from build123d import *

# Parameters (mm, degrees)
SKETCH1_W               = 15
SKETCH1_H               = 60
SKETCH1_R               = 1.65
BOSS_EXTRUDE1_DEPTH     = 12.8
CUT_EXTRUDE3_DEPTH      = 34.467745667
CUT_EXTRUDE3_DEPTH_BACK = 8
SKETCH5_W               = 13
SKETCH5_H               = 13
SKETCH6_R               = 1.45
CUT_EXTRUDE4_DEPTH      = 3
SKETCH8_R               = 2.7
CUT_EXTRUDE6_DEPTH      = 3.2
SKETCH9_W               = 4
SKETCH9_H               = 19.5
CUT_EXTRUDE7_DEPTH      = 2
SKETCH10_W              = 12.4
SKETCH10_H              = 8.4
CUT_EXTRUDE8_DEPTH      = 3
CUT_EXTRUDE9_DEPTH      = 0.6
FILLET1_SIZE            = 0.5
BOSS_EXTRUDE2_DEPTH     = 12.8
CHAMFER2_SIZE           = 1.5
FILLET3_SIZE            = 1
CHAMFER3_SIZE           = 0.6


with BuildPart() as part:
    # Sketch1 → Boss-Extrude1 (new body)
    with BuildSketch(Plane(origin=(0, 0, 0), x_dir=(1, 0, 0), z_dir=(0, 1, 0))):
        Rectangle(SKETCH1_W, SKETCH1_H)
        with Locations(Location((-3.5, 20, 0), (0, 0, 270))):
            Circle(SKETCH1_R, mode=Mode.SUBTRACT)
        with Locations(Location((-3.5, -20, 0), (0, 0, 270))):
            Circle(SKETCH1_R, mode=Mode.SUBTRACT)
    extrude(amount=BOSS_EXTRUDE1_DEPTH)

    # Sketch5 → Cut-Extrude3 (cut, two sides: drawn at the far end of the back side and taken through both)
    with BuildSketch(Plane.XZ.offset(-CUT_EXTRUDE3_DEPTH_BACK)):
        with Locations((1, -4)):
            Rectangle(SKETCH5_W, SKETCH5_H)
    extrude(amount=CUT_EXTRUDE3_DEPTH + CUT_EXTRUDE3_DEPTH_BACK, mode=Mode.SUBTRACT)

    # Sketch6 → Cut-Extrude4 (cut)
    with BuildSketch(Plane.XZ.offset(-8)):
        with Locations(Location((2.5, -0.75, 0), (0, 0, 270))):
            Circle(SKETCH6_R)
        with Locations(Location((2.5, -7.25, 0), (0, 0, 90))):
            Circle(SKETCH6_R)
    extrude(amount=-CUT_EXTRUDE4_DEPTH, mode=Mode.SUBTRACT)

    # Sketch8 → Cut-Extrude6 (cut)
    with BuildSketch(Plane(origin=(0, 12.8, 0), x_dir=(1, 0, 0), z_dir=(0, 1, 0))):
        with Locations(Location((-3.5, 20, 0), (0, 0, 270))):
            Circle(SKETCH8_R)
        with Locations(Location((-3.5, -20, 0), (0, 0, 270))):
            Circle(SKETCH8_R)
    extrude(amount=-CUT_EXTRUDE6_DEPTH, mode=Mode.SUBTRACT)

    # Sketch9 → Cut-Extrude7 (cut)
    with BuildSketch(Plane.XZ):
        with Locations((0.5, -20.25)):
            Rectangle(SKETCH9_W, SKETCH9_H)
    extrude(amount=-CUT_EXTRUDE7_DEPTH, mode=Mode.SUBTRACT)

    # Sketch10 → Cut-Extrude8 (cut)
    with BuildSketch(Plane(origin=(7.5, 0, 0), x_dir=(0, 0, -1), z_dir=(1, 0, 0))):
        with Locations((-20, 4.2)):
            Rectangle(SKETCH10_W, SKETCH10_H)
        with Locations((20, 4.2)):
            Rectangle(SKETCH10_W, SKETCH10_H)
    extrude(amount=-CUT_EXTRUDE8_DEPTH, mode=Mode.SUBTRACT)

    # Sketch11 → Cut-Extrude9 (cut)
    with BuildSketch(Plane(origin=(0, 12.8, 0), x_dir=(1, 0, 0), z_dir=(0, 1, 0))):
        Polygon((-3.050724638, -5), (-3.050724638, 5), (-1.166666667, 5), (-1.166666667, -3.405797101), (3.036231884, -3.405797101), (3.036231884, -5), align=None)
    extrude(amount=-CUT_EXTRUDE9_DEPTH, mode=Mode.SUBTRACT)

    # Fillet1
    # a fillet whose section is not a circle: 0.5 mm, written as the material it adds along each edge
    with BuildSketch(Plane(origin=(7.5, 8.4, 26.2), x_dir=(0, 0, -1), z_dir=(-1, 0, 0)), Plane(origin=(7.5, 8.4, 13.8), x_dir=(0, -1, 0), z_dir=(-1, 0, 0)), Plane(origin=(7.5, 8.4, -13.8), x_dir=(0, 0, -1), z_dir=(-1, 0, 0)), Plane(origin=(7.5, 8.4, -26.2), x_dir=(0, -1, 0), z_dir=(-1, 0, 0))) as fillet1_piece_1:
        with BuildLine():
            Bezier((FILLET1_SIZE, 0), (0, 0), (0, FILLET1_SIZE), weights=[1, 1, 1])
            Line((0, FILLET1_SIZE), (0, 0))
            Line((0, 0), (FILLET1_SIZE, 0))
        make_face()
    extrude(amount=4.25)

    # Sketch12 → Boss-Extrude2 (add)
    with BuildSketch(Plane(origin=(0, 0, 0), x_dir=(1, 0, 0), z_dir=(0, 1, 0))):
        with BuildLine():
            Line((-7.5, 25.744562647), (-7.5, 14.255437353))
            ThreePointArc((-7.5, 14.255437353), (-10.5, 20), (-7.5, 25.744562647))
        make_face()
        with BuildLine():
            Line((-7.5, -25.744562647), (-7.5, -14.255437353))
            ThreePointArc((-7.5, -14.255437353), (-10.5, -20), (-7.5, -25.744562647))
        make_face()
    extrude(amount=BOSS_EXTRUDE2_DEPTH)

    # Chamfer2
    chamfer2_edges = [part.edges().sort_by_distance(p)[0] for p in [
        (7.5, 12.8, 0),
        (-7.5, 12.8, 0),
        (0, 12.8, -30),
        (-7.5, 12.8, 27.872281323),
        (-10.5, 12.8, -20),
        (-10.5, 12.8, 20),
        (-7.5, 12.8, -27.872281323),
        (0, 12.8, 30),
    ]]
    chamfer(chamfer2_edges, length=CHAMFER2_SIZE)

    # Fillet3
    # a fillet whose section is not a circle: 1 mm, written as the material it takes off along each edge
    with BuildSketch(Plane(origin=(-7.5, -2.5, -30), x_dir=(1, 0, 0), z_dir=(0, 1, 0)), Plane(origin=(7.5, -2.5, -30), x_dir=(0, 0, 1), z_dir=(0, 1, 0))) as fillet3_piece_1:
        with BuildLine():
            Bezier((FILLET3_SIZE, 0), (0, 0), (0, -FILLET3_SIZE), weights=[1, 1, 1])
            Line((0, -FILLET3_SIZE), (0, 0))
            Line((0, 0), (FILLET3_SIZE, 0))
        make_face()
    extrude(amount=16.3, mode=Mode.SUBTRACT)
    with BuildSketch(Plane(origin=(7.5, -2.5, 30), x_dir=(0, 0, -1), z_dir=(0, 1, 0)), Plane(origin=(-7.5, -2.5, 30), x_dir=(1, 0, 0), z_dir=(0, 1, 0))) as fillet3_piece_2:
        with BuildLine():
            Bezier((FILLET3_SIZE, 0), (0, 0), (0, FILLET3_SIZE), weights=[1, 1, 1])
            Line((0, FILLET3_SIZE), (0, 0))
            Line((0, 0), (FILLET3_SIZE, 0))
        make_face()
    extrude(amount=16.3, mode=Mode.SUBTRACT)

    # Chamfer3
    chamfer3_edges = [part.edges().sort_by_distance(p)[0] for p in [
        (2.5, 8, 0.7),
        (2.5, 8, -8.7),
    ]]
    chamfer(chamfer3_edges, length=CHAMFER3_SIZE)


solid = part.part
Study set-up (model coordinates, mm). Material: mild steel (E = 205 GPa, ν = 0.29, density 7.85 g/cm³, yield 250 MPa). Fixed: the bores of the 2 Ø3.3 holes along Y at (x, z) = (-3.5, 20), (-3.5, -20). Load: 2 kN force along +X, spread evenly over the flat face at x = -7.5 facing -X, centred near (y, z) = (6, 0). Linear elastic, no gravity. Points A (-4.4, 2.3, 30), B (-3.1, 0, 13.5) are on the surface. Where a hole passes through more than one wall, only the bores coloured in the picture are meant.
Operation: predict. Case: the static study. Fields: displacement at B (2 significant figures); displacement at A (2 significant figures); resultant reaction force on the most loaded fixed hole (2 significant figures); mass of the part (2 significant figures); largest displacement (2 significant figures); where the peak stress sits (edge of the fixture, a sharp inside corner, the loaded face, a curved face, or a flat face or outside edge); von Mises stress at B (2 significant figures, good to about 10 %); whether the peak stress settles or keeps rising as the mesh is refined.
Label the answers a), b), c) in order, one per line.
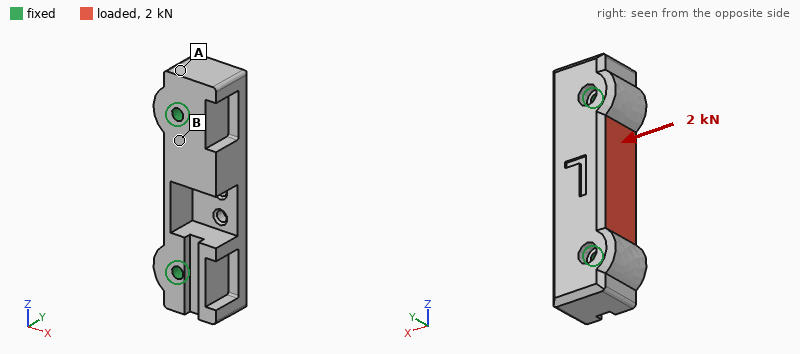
a) 1.9 µm
b) 1.7 µm
c) 1.0 kN
d) 74 g
e) 10 µm
f) edge of the fixture
g) 20 MPa
h) keeps rising
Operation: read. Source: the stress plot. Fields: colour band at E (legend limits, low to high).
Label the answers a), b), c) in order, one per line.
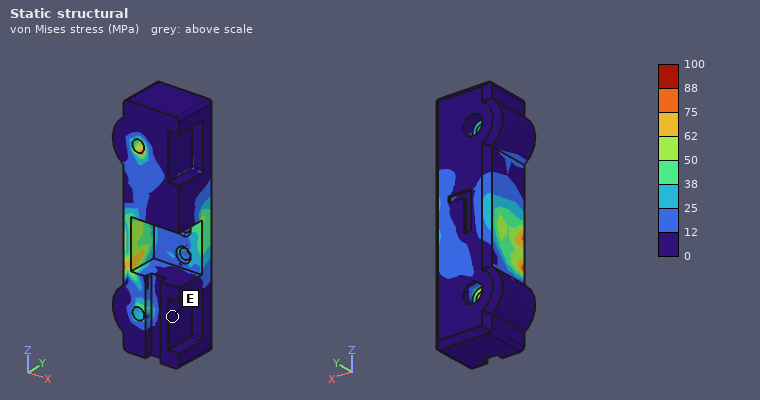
a) 0 to 12 MPa
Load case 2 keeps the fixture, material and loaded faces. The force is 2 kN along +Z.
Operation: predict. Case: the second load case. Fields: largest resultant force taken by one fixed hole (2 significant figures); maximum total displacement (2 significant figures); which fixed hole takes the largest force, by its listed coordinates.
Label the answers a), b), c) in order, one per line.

a) 1.1 kN
b) 1.5 µm
c) (-3.5, 20)
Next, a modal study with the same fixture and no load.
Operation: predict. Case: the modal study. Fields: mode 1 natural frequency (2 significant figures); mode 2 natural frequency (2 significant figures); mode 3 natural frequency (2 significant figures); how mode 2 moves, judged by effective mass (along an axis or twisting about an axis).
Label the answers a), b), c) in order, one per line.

a) 18 kHz
b) 22 kHz
c) 28 kHz
d) along Y
